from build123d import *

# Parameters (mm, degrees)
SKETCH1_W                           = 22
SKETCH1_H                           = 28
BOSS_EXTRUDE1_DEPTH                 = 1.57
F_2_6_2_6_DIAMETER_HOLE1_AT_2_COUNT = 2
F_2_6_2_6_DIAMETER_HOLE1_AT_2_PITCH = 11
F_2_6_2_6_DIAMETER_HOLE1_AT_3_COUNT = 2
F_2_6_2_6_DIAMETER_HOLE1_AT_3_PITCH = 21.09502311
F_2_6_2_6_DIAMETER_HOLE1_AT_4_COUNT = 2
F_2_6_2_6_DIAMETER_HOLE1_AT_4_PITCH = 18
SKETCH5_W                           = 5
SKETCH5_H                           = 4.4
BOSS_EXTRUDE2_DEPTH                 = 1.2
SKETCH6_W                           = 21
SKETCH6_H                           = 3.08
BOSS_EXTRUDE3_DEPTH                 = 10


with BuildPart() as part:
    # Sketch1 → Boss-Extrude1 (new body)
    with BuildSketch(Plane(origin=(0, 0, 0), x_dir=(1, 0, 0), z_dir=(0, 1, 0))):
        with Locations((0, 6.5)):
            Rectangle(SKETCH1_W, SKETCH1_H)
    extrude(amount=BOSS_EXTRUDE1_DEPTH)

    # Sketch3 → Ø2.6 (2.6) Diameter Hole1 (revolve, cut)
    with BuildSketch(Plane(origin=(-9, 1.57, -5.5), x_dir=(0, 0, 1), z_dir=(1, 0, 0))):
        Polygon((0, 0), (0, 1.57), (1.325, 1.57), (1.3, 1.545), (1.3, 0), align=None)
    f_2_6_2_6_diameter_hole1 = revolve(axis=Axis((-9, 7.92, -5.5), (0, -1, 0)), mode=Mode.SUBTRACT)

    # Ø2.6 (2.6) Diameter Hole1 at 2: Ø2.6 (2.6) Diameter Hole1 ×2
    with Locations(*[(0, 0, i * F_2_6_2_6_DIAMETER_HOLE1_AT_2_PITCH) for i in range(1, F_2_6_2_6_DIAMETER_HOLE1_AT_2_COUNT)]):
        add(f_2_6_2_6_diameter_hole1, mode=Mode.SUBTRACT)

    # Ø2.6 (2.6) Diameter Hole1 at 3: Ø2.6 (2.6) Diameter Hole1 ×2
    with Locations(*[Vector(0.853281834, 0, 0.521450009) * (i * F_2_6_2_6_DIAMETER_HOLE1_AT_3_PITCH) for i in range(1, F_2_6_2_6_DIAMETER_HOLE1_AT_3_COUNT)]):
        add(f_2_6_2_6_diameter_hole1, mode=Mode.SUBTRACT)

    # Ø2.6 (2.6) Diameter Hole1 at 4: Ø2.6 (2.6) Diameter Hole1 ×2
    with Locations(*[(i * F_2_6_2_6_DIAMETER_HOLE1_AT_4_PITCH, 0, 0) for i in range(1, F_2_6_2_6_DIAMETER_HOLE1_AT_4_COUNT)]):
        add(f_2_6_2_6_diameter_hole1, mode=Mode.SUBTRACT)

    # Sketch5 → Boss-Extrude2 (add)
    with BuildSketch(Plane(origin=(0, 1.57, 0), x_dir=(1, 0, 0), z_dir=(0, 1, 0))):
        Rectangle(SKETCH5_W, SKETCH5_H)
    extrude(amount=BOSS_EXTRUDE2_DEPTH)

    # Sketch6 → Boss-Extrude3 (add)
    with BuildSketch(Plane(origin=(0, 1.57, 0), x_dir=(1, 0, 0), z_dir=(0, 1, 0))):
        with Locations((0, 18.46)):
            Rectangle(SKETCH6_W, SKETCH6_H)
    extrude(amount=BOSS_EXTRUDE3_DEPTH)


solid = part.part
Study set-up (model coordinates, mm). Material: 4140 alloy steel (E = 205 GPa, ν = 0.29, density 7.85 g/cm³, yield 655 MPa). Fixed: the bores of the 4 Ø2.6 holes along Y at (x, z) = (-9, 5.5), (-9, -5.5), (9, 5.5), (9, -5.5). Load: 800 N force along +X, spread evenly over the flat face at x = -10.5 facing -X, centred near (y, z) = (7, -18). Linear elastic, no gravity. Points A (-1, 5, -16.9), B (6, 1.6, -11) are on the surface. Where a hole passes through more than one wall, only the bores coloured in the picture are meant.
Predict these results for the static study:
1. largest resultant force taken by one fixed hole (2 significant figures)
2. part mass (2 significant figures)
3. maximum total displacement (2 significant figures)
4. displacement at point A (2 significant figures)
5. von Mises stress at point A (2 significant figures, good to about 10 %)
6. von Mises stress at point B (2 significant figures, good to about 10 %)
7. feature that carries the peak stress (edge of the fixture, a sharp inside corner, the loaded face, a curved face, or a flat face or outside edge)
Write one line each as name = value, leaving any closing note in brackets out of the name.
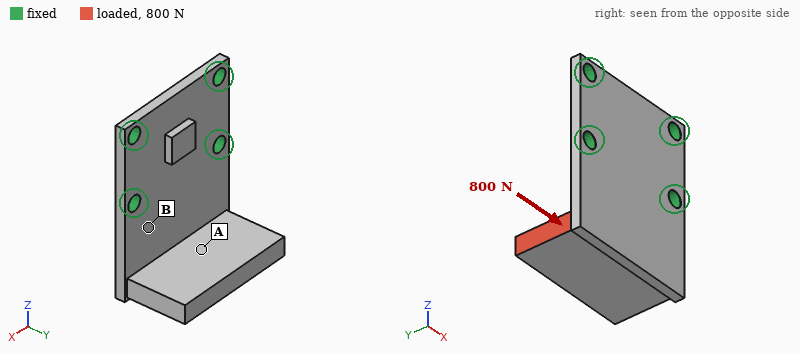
largest resultant force taken by one fixed hole = 710 N
part mass = 13 g
maximum total displacement = 0.12 mm
displacement at point A = 0.040 mm
von Mises stress at point A = 76 MPa
von Mises stress at point B = 250 MPa
feature that carries the peak stress = edge of the fixture
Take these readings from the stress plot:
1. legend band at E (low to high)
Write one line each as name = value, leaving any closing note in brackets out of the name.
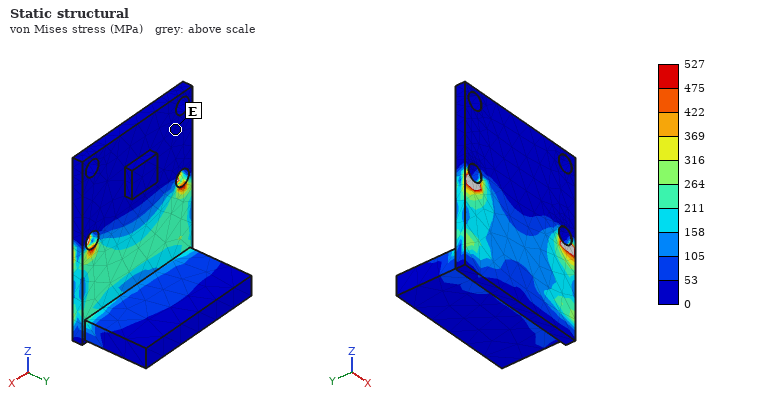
legend band at E = 0 to 53 MPa
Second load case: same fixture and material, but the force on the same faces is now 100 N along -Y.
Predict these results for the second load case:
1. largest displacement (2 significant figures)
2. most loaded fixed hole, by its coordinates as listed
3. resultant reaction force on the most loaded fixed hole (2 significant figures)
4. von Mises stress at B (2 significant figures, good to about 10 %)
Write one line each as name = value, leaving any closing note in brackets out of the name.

largest displacement = 0.10 mm
most loaded fixed hole, by its coordinates as listed = (-9, -5.5)
resultant reaction force on the most loaded fixed hole = 130 N
von Mises stress at B = 70 MPa
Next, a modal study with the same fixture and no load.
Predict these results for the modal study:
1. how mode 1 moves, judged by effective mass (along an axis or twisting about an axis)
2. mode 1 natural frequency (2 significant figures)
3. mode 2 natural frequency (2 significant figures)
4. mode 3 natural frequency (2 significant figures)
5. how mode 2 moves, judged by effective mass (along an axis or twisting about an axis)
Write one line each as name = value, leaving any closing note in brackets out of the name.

how mode 1 moves, judged by effective mass = along Y
mode 1 natural frequency = 2300 Hz
mode 2 natural frequency = 5600 Hz
mode 3 natural frequency = 8900 Hz
how mode 2 moves, judged by effective mass = along X
